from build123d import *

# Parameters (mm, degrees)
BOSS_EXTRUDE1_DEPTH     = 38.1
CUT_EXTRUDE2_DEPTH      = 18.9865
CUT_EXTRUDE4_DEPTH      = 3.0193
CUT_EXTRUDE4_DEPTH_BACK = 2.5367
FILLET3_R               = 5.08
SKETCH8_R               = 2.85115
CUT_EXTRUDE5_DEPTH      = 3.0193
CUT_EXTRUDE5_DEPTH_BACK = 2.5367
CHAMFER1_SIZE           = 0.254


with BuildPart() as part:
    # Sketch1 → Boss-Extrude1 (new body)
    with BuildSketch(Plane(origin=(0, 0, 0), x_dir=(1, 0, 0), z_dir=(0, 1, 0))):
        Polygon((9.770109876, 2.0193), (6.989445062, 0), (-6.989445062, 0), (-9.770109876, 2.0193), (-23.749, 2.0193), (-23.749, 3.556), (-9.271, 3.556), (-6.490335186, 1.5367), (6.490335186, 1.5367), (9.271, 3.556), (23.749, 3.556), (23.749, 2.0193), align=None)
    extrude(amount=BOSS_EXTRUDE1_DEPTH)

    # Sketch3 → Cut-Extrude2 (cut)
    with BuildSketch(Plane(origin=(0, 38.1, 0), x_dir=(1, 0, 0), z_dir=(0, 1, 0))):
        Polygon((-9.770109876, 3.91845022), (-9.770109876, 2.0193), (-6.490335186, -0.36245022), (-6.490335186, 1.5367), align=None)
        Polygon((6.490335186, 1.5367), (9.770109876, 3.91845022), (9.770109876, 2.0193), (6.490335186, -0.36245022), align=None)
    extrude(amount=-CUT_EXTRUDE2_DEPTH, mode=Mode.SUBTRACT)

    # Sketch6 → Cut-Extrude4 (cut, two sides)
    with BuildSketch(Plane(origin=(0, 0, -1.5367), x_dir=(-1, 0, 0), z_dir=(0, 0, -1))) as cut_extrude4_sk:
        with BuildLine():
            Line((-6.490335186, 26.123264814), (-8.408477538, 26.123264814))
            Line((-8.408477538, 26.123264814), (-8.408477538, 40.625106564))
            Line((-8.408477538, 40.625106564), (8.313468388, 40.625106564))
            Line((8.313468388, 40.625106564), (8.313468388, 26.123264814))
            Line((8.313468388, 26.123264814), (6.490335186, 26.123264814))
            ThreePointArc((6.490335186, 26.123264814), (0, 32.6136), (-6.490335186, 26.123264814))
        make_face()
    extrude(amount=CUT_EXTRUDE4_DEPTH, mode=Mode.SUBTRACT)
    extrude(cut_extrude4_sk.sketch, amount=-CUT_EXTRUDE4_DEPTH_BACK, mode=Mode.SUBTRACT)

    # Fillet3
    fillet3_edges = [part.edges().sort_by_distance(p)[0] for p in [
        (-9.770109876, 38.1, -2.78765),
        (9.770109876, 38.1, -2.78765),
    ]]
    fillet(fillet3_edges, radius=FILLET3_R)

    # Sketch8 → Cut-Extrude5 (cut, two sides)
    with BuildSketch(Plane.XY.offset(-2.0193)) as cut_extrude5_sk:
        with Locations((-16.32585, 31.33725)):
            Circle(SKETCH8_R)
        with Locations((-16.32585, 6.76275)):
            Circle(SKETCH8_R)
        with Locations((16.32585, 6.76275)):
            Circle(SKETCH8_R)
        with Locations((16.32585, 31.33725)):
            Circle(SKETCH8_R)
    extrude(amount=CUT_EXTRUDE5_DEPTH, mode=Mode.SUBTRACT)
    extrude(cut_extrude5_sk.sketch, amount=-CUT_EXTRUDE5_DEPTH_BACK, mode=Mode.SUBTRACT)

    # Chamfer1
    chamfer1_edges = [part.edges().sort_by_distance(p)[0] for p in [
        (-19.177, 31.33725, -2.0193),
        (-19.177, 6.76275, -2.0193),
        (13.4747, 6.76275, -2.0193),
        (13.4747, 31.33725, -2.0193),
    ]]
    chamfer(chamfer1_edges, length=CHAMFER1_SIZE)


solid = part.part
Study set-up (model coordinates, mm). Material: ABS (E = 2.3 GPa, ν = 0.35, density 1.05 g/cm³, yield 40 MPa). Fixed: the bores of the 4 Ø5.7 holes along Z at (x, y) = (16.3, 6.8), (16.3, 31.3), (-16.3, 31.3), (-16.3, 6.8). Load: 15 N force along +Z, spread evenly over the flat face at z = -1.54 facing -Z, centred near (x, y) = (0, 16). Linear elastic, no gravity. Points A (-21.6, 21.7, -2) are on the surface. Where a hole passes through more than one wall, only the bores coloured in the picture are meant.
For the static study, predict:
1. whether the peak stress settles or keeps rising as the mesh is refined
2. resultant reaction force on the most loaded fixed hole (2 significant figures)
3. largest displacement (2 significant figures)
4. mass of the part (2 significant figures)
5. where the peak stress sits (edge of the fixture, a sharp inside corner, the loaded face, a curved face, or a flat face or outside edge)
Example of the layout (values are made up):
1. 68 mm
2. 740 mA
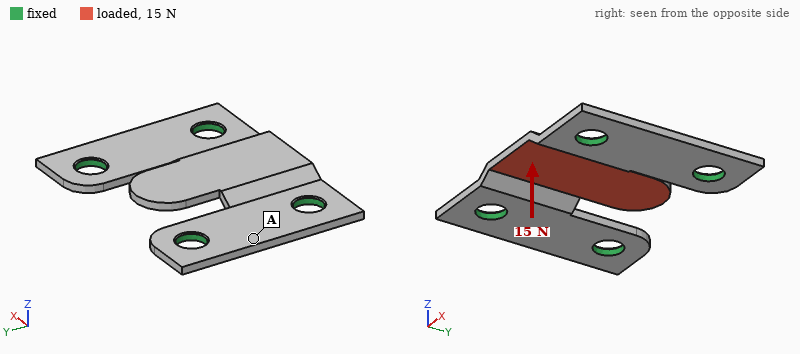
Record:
1. keeps rising
2. 18 N
3. 0.65 mm
4. 2.4 g
5. a sharp inside corner
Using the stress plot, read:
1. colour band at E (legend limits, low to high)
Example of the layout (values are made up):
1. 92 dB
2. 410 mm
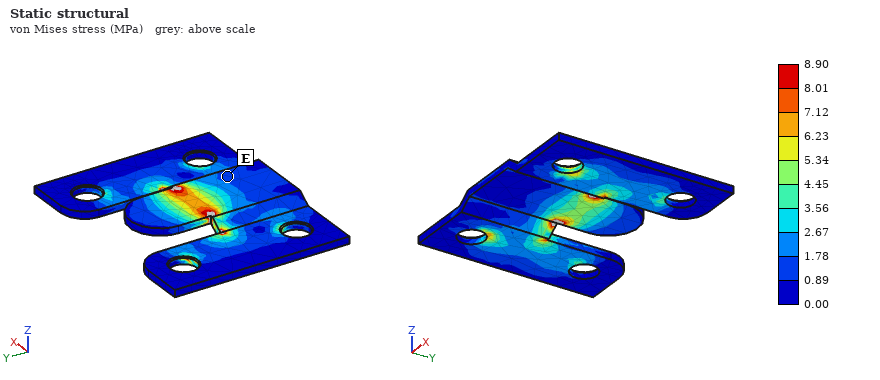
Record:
1. 0.89 to 1.78 MPa
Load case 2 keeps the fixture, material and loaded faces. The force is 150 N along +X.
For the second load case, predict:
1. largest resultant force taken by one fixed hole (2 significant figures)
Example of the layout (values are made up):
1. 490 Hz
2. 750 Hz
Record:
1. 73 N
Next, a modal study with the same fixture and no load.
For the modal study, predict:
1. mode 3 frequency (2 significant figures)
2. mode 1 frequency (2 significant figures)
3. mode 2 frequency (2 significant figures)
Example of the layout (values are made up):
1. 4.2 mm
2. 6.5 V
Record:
1. 3800 Hz
2. 1200 Hz
3. 3700 Hz
